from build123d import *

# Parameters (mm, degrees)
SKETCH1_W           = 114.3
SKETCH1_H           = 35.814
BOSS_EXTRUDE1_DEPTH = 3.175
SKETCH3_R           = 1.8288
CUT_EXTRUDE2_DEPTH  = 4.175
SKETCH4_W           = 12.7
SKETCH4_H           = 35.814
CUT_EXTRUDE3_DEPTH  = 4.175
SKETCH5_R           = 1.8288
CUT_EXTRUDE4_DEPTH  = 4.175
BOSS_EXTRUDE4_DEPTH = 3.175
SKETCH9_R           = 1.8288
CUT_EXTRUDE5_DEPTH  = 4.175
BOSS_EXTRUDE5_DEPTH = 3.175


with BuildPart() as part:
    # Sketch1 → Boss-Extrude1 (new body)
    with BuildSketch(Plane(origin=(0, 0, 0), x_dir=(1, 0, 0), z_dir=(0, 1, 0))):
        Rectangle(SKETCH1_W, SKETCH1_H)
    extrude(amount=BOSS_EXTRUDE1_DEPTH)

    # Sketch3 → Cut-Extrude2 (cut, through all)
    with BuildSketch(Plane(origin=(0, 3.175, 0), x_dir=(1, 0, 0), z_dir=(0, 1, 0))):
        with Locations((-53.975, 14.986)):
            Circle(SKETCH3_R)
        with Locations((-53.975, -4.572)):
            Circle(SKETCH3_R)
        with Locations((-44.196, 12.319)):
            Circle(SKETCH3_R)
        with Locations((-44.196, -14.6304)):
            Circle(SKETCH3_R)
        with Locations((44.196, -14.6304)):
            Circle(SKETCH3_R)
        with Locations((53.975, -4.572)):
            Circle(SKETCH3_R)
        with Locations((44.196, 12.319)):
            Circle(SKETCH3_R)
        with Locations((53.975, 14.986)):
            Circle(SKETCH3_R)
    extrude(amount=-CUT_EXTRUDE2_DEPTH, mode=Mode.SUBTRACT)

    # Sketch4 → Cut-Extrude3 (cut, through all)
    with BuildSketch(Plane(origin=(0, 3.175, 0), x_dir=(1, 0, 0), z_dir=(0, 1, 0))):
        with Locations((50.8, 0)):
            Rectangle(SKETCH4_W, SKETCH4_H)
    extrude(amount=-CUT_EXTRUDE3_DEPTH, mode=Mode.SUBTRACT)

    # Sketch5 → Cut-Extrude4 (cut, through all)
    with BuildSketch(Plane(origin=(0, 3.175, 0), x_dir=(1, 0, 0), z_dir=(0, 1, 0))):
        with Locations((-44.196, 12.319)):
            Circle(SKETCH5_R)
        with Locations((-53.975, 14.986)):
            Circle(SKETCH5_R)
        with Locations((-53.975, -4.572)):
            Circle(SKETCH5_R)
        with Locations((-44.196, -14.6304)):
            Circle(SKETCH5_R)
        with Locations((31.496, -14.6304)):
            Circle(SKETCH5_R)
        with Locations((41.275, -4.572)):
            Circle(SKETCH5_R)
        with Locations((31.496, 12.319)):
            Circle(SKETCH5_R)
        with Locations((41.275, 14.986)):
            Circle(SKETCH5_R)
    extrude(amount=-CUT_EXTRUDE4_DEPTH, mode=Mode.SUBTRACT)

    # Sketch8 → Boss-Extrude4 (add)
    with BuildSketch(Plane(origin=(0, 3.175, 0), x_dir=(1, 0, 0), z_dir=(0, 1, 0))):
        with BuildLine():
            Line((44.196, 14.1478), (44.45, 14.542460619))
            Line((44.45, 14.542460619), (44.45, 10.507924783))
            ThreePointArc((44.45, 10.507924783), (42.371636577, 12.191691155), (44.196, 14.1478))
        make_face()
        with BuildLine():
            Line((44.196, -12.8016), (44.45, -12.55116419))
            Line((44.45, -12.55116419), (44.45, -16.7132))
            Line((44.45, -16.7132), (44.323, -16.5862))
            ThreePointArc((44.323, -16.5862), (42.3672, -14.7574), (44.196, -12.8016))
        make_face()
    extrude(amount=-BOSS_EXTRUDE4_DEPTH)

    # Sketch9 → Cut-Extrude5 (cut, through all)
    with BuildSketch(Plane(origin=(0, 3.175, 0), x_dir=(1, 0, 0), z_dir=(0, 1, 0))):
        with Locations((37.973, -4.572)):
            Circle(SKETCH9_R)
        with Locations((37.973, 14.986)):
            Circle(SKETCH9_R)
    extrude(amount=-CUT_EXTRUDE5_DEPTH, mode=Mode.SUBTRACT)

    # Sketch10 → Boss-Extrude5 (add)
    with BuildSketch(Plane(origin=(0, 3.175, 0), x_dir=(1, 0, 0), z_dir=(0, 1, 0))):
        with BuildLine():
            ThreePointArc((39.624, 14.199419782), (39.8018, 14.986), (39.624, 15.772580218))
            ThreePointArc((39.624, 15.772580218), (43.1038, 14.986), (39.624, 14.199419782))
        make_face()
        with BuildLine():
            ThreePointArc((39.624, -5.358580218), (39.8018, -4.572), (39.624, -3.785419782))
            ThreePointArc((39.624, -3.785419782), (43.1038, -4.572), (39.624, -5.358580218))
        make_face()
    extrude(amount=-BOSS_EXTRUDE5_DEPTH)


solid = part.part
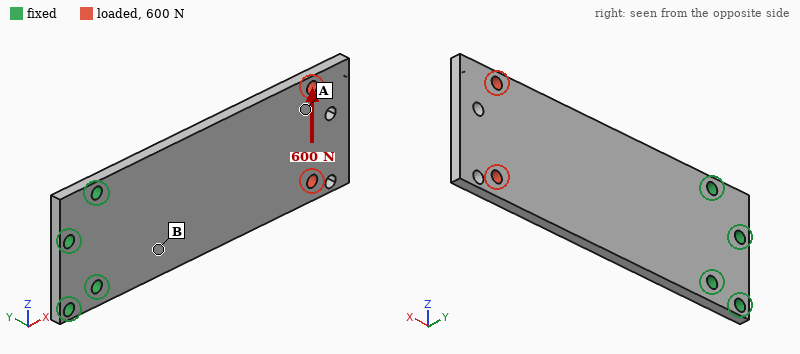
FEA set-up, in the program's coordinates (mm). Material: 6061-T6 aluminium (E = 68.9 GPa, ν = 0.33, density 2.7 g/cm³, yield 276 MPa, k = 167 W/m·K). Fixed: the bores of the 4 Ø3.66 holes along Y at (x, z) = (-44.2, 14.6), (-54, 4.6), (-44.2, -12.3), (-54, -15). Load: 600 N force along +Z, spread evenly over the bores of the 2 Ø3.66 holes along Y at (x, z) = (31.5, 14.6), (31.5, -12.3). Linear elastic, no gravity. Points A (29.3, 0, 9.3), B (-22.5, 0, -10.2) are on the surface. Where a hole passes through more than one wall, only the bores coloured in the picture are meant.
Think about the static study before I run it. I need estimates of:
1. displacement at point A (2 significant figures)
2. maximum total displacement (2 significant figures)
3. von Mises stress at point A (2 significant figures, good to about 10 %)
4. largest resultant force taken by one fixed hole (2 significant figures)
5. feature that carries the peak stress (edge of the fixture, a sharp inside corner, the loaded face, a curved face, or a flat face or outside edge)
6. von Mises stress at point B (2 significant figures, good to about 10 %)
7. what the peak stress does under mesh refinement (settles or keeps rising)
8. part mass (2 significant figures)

0.12 mm
0.15 mm
11 MPa
1.5 kN
edge of the fixture
29 MPa
keeps rising
30 g
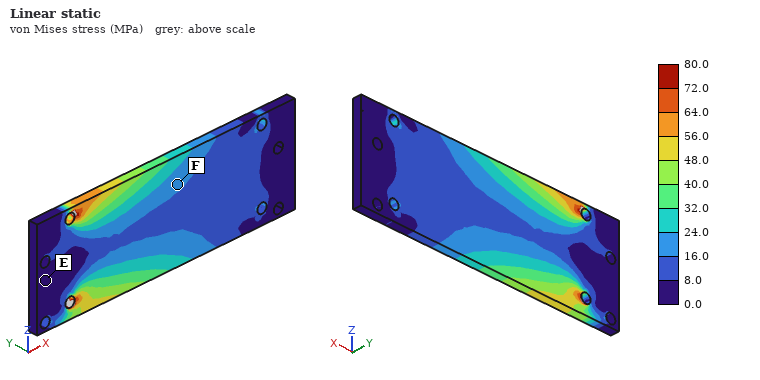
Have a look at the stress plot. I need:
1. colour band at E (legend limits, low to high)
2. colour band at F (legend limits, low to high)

0.0 to 8.0 MPa
16.0 to 24.0 MPa
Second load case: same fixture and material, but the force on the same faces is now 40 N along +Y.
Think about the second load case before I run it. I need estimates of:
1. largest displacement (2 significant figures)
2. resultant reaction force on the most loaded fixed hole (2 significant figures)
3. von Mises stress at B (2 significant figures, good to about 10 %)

1.1 mm
78 N
35 MPa
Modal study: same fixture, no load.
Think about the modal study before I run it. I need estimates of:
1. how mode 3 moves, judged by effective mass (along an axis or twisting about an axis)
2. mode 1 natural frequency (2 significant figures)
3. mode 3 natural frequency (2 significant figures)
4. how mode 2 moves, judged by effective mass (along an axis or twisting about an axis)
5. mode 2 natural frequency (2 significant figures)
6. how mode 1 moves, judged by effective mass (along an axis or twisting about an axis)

along Y
340 Hz
2100 Hz
twisting about X
1700 Hz
along Y
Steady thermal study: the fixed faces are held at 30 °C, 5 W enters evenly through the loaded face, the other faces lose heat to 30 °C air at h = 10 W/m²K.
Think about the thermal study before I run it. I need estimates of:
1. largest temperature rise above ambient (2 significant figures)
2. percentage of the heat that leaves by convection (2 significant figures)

20 K
15 %
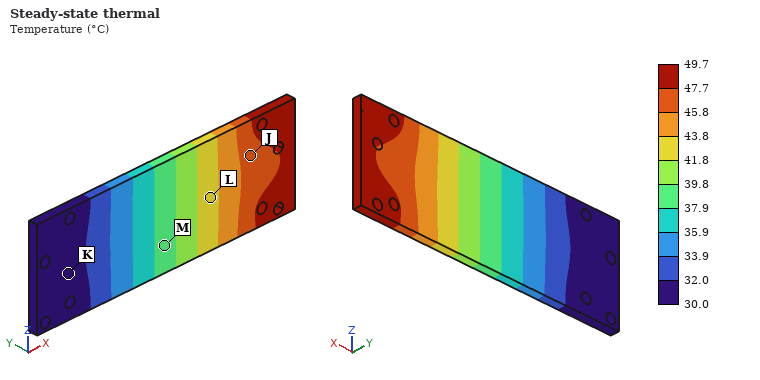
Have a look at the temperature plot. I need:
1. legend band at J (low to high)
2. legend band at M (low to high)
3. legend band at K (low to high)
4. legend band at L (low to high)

45.8 to 47.7 °C
37.9 to 39.8 °C
30.0 to 32.0 °C
41.8 to 43.8 °C
